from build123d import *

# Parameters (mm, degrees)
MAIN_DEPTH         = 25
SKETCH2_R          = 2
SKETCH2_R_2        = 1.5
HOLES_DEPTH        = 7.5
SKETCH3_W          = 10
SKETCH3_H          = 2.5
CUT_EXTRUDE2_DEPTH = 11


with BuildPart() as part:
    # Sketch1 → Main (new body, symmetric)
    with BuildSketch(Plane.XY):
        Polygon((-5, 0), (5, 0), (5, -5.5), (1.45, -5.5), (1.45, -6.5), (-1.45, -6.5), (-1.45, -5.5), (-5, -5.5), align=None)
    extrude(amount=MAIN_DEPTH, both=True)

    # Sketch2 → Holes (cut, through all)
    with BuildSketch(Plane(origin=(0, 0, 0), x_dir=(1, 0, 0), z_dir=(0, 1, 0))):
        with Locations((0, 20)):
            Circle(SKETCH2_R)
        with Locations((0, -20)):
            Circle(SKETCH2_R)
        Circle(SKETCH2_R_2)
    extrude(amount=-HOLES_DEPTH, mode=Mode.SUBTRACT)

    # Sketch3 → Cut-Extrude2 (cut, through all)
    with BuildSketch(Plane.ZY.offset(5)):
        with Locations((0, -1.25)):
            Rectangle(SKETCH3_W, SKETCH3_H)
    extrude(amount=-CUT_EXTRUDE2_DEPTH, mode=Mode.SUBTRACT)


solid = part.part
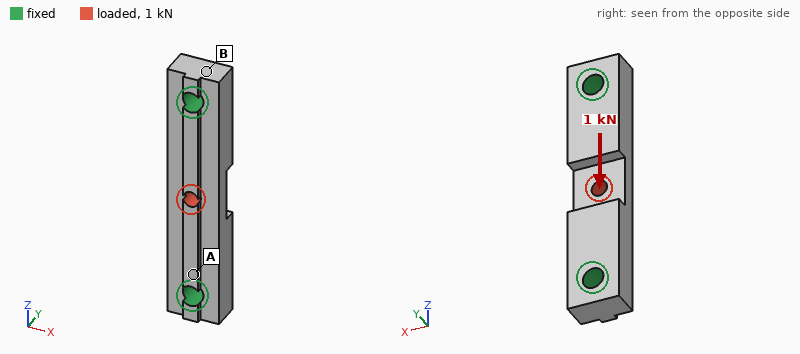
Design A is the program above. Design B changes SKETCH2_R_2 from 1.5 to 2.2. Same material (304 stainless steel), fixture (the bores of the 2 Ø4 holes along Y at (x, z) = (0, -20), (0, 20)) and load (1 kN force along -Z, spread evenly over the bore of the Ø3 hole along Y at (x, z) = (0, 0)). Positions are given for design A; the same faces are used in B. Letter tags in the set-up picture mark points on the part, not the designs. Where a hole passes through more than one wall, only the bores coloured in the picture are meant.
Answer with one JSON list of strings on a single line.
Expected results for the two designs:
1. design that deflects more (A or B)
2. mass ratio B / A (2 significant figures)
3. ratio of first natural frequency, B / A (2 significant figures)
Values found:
["A", "0.99", "1.0"]
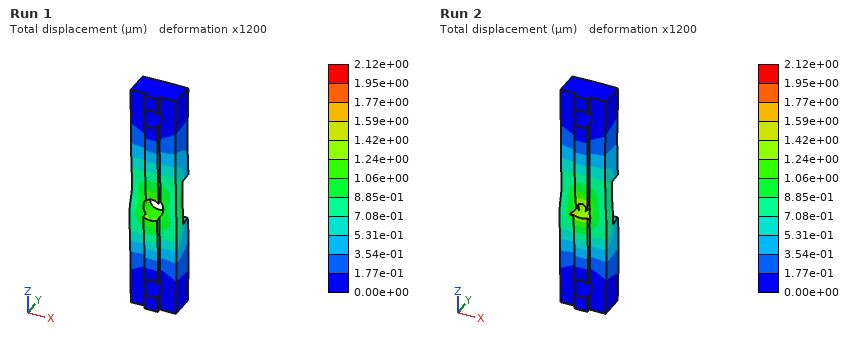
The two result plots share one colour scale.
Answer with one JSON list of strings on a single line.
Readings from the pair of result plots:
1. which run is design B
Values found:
["Run 1"]
